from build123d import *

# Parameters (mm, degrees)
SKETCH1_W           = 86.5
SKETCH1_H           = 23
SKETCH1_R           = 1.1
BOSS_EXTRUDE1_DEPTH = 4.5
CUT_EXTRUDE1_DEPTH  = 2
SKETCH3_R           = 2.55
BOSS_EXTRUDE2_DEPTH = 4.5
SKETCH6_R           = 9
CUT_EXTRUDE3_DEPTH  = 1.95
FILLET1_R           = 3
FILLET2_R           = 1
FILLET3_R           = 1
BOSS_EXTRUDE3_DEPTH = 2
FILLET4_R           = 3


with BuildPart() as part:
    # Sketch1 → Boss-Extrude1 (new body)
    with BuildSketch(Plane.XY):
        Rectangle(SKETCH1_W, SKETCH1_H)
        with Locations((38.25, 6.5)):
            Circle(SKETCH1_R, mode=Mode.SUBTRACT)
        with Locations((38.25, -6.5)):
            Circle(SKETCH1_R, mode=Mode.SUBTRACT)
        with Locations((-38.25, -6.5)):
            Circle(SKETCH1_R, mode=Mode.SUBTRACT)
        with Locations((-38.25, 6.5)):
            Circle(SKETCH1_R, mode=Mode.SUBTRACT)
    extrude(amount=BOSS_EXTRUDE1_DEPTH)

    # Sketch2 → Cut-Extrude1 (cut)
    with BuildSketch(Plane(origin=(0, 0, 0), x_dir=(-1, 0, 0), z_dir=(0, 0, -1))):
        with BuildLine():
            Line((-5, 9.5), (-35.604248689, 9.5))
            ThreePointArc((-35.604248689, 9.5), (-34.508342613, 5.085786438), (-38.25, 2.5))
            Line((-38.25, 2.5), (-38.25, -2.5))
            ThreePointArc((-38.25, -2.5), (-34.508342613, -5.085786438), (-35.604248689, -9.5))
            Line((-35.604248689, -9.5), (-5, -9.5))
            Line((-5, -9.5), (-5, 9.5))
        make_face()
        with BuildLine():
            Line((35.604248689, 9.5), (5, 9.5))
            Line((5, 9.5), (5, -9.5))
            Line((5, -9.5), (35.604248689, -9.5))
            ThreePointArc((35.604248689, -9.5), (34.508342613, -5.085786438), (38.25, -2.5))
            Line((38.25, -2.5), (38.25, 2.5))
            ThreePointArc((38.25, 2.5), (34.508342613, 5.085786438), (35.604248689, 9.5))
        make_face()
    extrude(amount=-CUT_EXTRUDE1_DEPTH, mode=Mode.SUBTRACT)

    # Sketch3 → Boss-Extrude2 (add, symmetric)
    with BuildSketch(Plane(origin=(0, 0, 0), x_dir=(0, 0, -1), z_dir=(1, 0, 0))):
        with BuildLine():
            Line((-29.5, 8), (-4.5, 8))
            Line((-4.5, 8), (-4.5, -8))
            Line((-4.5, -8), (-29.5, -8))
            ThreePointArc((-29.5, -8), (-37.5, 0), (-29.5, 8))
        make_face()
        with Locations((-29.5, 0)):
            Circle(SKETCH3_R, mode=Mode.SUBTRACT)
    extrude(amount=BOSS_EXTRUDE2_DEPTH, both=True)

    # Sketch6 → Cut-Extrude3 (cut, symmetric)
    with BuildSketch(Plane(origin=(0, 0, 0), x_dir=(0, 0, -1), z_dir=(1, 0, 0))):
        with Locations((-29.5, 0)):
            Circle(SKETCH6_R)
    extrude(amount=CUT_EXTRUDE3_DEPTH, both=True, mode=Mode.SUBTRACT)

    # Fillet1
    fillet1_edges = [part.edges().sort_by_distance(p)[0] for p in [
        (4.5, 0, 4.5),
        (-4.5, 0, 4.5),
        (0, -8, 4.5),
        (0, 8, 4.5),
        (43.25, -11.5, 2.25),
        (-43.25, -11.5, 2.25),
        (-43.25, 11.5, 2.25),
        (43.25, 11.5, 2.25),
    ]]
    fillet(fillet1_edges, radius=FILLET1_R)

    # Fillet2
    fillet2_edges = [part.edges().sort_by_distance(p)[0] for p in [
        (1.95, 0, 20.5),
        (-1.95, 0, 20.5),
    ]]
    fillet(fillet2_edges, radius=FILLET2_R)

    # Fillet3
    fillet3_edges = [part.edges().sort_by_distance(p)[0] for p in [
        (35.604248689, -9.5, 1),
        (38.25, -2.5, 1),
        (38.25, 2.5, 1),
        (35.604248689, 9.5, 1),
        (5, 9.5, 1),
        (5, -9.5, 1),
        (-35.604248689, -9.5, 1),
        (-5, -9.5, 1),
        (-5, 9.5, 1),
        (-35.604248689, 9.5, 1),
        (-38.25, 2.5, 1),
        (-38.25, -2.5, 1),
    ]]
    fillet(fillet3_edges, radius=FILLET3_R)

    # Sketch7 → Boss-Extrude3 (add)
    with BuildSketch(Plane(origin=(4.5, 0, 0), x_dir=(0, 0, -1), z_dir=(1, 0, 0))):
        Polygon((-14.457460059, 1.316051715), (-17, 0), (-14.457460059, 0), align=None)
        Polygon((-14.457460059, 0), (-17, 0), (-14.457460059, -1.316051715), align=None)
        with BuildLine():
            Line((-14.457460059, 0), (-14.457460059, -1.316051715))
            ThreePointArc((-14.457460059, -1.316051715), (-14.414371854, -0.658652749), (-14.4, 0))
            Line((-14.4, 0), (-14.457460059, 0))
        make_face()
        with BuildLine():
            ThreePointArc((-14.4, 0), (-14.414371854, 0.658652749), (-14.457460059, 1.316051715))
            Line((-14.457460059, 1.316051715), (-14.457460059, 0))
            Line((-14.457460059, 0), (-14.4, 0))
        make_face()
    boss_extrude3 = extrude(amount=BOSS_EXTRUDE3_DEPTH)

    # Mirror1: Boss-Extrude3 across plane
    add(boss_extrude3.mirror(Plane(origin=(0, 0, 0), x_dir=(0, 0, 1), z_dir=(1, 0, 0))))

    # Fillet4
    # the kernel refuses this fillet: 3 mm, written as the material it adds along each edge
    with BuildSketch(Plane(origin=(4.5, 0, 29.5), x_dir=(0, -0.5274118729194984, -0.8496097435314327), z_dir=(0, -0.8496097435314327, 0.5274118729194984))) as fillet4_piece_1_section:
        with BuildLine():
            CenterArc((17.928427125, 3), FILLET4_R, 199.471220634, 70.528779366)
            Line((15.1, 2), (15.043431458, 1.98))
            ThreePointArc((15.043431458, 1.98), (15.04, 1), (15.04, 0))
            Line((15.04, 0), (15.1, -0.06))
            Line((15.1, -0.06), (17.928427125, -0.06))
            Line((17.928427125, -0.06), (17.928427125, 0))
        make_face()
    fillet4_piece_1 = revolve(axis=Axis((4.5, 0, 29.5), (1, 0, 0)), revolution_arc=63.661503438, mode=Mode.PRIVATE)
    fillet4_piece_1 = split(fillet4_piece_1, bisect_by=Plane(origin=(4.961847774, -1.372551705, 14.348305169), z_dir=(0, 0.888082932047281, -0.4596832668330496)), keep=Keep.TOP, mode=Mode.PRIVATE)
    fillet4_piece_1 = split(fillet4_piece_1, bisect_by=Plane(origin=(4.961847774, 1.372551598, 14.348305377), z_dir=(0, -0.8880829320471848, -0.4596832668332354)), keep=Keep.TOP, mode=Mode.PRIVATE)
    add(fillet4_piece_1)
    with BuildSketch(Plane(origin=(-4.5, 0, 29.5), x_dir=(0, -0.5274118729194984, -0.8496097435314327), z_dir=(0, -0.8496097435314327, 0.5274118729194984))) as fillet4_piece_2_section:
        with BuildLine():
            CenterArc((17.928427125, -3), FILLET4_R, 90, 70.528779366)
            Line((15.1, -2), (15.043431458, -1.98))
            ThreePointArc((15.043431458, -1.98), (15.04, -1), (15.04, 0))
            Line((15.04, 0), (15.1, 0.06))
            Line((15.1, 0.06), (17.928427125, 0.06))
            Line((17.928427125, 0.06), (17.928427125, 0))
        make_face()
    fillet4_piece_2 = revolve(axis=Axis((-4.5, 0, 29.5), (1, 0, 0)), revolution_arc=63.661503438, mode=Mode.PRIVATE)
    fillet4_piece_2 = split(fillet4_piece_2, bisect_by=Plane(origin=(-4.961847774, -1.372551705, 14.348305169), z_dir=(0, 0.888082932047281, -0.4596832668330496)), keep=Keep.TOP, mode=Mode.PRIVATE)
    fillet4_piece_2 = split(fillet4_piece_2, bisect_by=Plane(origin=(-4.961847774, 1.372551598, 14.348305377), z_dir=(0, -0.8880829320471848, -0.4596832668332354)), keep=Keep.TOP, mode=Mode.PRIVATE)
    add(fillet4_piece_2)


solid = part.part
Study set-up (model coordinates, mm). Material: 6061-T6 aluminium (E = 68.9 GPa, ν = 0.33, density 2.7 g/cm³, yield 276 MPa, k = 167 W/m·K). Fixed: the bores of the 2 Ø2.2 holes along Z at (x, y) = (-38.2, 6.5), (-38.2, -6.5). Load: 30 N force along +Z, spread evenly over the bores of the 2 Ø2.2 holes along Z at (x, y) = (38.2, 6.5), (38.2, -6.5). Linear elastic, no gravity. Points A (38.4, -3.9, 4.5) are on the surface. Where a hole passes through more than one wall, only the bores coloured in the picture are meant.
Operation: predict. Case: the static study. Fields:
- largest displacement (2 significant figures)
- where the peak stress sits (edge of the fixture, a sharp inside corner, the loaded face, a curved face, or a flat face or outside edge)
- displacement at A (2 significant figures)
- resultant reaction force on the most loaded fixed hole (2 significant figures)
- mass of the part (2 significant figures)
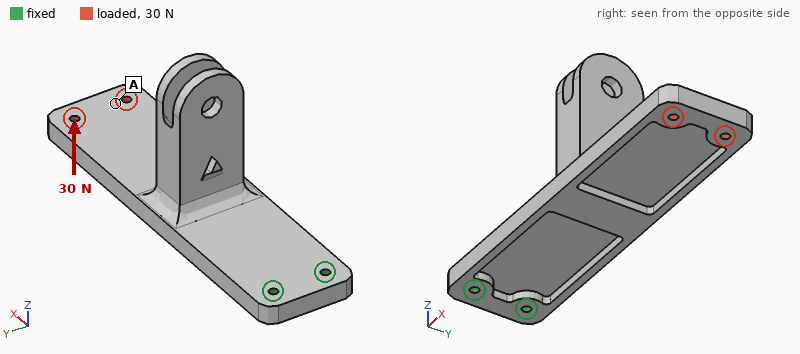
0.92 mm
a curved face
0.84 mm
42 N
28 g
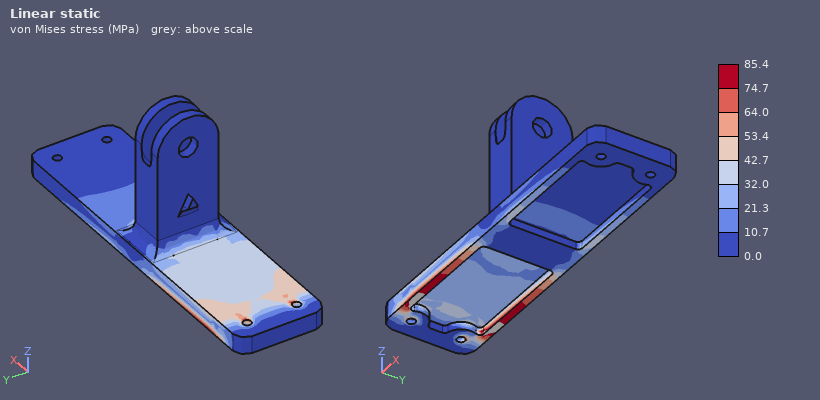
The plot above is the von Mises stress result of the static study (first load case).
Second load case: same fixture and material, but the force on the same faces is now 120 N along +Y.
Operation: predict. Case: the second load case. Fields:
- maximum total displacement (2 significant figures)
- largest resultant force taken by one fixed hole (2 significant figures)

0.11 mm
640 N
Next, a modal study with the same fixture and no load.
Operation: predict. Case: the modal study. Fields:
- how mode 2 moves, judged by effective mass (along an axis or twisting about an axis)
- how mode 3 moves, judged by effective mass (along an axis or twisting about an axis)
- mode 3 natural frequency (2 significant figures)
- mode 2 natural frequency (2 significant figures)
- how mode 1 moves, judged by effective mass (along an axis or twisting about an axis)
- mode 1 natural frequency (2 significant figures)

along Y
along Z
2000 Hz
1200 Hz
along Z
360 Hz
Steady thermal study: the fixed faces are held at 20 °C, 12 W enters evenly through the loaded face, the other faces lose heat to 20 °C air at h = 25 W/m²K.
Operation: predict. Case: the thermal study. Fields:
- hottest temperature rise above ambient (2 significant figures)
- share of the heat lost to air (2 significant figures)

58 K
38 %
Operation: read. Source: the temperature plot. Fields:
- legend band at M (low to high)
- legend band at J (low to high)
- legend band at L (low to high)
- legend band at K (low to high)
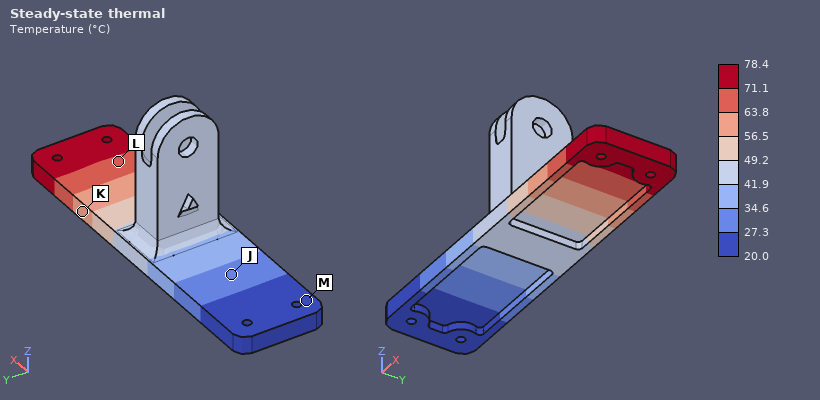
20.0 to 27.3 °C
27.3 to 34.6 °C
63.8 to 71.1 °C
56.5 to 63.8 °C
